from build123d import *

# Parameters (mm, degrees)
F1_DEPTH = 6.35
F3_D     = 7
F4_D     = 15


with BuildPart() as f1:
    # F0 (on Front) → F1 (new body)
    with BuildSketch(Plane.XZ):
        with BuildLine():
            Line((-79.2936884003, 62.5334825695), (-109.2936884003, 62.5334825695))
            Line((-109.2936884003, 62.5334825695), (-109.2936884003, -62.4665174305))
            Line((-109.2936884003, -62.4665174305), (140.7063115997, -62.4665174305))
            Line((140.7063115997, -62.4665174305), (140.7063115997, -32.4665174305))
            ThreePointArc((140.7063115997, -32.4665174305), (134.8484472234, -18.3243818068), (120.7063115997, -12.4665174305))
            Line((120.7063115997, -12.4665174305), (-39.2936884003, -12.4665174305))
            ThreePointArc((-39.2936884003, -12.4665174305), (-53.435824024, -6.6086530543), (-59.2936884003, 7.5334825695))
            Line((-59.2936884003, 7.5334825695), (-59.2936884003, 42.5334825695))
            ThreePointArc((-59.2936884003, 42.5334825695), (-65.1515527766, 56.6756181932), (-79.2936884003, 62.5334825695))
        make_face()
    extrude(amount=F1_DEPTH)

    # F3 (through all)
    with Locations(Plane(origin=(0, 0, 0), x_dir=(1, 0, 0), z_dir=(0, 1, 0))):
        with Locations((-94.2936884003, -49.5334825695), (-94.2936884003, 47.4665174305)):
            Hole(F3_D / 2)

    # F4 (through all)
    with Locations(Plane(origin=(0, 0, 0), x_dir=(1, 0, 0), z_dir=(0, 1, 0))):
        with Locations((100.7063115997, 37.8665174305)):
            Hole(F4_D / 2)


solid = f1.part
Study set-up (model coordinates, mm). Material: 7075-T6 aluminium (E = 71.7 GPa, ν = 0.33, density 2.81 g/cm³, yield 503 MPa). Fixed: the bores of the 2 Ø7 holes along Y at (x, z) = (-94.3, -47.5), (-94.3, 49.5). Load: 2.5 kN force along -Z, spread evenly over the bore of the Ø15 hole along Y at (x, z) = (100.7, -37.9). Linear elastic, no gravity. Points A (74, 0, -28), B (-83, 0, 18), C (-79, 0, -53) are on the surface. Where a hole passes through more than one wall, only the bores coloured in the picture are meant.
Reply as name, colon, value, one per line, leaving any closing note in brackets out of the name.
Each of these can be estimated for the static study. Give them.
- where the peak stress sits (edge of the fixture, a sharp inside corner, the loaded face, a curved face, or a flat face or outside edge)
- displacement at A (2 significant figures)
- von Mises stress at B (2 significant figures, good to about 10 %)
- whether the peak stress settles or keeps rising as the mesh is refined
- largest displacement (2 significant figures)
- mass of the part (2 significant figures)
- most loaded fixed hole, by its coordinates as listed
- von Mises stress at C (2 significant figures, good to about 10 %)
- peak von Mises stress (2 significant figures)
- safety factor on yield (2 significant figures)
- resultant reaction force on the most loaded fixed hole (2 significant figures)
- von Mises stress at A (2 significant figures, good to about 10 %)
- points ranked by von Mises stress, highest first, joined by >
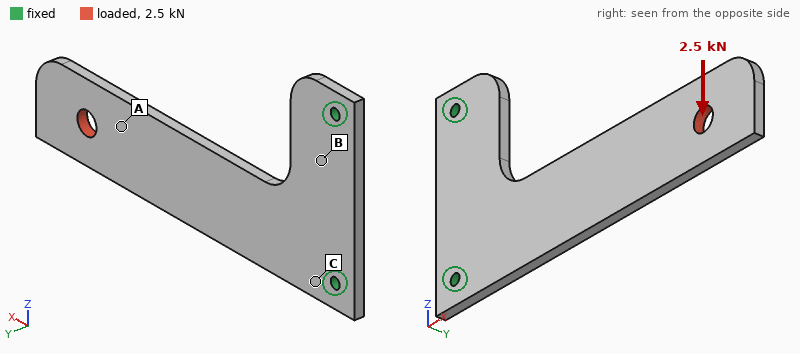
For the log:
where the peak stress sits: a curved face
displacement at A: 0.87 mm
von Mises stress at B: 42 MPa
whether the peak stress settles or keeps rising as the mesh is refined: settles
largest displacement: 1.5 mm
mass of the part: 280 g
most loaded fixed hole, by its coordinates as listed: (-94.3, 49.5)
von Mises stress at C: 67 MPa
peak von Mises stress: 210 MPa
safety factor on yield: 2.4
resultant reaction force on the most loaded fixed hole: 6.6 kN
von Mises stress at A: 20 MPa
points ranked by von Mises stress, highest first, joined by >: C > B > A
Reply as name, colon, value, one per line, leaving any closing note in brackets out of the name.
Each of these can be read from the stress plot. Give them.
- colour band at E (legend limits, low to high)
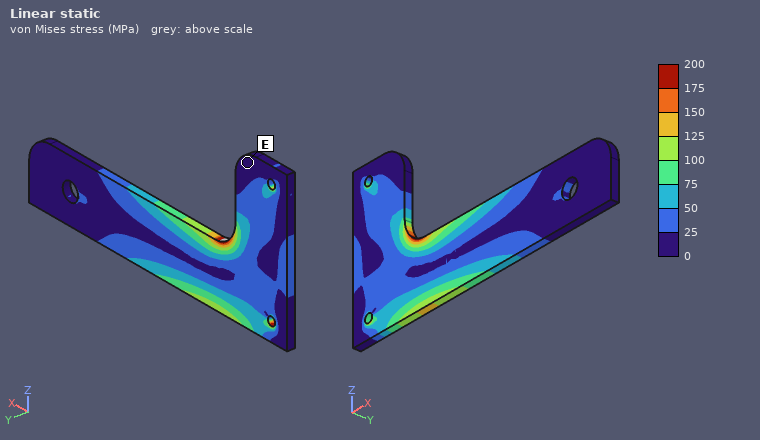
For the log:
colour band at E: 0 to 25 MPa
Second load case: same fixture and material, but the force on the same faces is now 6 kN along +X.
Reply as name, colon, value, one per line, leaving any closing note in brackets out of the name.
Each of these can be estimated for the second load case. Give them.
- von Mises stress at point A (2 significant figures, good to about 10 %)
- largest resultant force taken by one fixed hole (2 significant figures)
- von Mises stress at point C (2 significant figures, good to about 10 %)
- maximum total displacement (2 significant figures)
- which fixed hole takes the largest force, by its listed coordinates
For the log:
von Mises stress at point A: 20 MPa
largest resultant force taken by one fixed hole: 5.4 kN
von Mises stress at point C: 27 MPa
maximum total displacement: 63 µm
which fixed hole takes the largest force, by its listed coordinates: (-94.3, -47.5)
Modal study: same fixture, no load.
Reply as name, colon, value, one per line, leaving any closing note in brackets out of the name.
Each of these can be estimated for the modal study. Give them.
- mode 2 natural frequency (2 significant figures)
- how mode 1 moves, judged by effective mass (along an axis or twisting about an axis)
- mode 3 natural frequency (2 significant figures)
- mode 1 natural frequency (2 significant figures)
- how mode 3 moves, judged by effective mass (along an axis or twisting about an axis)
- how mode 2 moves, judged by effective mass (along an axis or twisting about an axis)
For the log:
mode 2 natural frequency: 610 Hz
how mode 1 moves, judged by effective mass: along Y
mode 3 natural frequency: 830 Hz
mode 1 natural frequency: 100 Hz
how mode 3 moves, judged by effective mass: along Z
how mode 2 moves, judged by effective mass: along Y
